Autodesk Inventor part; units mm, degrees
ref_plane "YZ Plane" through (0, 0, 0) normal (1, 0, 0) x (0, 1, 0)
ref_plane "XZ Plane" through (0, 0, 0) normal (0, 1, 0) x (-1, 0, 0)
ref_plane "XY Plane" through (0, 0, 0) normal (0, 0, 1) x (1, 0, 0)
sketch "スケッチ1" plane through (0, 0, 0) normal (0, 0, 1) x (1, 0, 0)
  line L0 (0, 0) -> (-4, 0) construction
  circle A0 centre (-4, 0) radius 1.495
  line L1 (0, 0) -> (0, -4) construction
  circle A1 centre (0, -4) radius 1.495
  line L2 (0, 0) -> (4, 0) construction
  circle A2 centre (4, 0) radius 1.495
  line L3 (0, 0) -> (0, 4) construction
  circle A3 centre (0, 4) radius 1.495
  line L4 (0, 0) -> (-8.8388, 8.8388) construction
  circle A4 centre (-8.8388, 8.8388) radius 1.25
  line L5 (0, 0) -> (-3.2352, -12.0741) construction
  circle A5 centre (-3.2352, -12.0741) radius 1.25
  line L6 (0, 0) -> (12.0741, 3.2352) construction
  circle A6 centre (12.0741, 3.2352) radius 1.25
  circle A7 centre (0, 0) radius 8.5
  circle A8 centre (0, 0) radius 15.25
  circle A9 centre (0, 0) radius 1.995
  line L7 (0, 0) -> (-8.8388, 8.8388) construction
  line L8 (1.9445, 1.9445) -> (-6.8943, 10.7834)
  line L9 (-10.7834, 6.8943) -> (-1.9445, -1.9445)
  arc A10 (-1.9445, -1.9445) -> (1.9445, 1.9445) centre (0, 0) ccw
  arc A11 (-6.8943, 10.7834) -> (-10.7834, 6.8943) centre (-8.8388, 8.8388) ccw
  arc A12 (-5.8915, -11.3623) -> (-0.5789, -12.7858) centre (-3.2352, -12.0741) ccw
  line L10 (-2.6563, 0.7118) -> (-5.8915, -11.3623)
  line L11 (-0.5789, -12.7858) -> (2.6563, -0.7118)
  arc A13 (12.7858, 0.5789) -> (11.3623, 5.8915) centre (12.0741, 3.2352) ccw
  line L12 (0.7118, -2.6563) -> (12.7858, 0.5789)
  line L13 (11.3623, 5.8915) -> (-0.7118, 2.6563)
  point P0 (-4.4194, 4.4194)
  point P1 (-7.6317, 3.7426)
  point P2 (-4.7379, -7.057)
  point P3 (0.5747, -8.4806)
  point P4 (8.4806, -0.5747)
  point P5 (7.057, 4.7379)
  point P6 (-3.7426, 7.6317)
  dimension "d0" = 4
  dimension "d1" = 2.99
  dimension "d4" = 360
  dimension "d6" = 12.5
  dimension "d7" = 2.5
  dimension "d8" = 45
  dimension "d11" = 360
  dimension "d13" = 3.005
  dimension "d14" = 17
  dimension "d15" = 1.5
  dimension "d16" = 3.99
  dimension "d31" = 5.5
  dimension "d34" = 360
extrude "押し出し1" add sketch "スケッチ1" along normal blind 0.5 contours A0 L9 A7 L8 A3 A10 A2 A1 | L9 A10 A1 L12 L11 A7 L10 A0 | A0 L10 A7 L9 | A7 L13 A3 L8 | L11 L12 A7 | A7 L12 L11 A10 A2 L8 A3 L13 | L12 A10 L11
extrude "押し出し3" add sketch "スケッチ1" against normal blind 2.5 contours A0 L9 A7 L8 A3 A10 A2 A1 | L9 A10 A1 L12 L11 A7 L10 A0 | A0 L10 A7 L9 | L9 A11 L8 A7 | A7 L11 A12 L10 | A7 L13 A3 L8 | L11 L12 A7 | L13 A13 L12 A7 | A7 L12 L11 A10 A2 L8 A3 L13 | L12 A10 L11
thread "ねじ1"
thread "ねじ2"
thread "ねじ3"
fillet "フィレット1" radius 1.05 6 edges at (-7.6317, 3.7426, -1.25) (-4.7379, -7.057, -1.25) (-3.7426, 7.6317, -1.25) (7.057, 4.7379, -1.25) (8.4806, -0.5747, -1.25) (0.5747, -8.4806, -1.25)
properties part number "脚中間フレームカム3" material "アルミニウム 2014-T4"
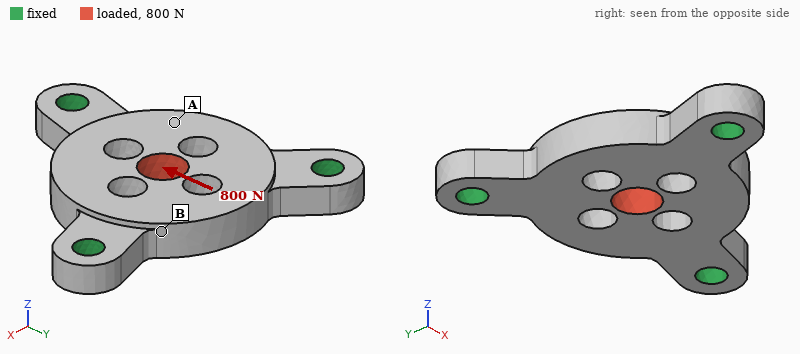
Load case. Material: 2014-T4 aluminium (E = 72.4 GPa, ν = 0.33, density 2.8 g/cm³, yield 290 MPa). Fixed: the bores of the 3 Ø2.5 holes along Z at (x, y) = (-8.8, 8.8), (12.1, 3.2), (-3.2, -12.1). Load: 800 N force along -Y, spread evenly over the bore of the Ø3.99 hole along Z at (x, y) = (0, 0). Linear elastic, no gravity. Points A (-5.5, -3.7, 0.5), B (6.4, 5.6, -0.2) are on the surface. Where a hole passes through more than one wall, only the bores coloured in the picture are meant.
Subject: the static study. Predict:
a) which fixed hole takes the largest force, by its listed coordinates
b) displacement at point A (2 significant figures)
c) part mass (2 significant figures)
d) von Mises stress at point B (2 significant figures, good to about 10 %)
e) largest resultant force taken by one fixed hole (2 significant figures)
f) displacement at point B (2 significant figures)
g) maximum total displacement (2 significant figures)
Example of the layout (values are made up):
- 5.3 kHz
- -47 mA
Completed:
- (-3.2, -12.1)
- 2.2 µm
- 2.2 g
- 25 MPa
- 380 N
- 5.2 µm
- 9.4 µm
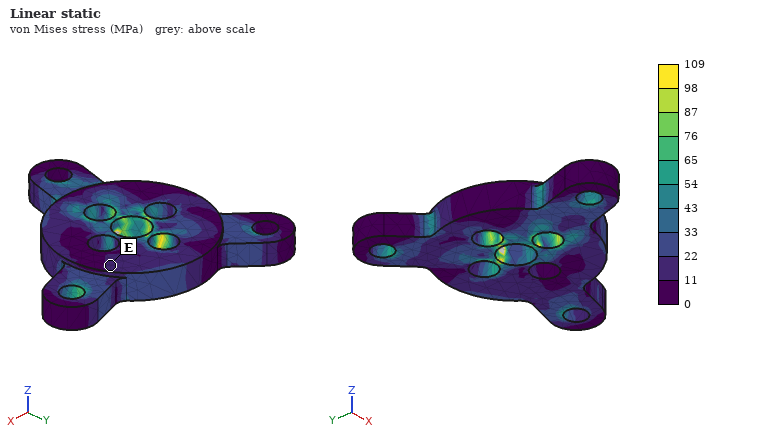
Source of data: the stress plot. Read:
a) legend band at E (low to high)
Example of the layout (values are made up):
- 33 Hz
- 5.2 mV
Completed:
- 11 to 22 MPa
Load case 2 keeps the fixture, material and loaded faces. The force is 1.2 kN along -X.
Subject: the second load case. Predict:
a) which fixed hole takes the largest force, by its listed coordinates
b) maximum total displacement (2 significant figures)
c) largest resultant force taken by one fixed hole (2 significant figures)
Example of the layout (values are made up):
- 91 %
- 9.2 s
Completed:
- (12.1, 3.2)
- 14 µm
- 570 N
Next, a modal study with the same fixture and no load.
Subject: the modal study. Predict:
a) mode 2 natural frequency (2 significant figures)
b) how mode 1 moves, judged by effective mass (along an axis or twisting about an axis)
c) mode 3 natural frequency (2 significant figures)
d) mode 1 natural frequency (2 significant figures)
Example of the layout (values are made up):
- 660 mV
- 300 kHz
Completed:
- 33 kHz
- along Z
- 33 kHz
- 25 kHz
